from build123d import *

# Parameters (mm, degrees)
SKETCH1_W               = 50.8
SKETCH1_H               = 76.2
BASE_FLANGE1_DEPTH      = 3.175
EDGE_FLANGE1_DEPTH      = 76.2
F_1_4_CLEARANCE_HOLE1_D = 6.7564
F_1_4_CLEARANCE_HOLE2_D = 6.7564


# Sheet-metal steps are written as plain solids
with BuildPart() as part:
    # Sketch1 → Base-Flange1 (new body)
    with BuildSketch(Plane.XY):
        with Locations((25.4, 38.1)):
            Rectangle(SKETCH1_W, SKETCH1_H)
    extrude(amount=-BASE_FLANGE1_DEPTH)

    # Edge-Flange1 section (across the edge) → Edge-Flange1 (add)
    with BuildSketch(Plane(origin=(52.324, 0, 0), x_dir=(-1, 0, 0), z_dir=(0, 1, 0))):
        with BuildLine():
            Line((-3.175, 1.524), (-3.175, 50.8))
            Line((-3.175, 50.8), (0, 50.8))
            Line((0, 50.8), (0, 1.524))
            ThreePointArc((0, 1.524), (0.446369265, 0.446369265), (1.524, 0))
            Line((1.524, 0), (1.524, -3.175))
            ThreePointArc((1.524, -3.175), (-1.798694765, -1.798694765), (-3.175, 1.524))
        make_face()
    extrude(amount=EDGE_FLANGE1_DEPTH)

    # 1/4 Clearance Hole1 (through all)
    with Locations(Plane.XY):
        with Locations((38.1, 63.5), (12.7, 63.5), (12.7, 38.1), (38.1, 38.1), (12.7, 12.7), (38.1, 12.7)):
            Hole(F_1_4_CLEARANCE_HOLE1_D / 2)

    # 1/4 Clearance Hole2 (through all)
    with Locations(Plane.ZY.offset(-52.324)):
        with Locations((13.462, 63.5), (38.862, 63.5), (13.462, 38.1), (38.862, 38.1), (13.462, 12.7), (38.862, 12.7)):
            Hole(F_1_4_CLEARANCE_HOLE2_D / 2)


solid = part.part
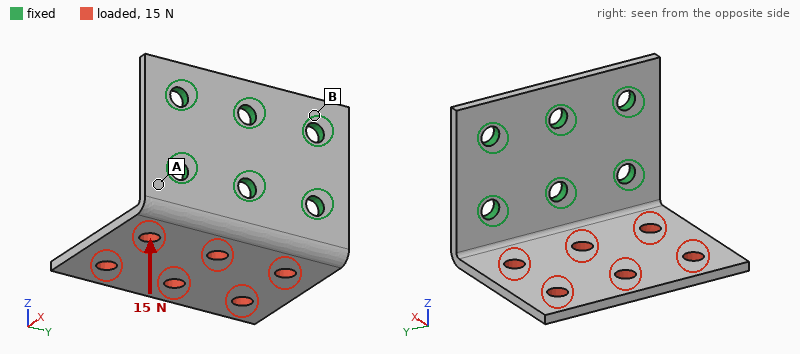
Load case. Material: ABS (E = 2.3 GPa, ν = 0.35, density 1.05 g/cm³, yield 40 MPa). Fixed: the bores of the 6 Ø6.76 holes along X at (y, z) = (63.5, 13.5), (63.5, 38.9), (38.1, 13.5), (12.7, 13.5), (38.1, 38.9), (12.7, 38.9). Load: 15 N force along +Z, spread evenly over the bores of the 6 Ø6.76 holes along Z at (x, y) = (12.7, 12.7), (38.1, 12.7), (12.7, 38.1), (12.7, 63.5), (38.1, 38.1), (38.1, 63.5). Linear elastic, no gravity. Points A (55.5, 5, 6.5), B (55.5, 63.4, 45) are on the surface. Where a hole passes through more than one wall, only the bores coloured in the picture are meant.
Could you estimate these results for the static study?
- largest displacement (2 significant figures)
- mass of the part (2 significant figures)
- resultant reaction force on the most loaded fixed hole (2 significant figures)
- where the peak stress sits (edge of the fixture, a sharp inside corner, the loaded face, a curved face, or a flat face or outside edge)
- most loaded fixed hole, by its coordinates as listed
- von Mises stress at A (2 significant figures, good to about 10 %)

1.2 mm
25 g
5.3 N
a flat face or outside edge
(38.1, 13.5)
2.7 MPa
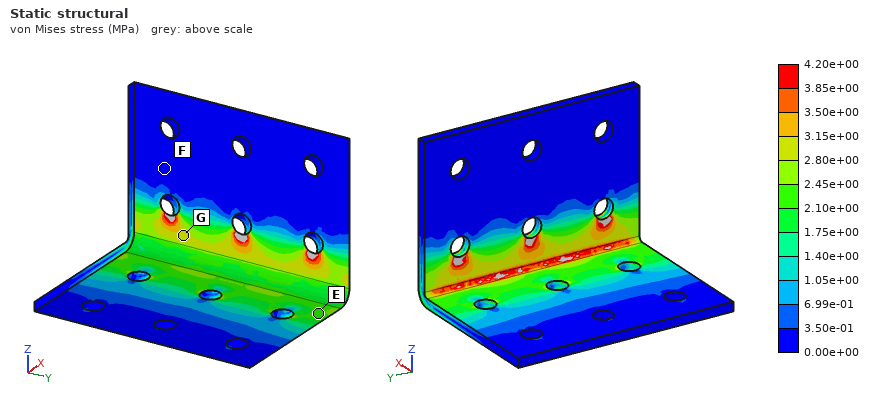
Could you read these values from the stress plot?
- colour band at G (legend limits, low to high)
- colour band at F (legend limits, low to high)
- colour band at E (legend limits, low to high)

2.80e+00 to 3.15e+00 MPa
0.00e+00 to 3.50e-01 MPa
2.10e+00 to 2.45e+00 MPa
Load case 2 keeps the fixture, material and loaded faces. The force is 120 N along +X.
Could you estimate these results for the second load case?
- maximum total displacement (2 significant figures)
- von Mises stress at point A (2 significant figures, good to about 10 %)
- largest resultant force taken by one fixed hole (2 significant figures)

1.2 mm
6.0 MPa
43 N
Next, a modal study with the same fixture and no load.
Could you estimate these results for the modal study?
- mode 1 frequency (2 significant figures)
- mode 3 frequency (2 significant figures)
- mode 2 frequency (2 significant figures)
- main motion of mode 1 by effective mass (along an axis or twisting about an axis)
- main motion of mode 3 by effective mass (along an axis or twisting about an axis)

200 Hz
810 Hz
410 Hz
along Z
along Y
